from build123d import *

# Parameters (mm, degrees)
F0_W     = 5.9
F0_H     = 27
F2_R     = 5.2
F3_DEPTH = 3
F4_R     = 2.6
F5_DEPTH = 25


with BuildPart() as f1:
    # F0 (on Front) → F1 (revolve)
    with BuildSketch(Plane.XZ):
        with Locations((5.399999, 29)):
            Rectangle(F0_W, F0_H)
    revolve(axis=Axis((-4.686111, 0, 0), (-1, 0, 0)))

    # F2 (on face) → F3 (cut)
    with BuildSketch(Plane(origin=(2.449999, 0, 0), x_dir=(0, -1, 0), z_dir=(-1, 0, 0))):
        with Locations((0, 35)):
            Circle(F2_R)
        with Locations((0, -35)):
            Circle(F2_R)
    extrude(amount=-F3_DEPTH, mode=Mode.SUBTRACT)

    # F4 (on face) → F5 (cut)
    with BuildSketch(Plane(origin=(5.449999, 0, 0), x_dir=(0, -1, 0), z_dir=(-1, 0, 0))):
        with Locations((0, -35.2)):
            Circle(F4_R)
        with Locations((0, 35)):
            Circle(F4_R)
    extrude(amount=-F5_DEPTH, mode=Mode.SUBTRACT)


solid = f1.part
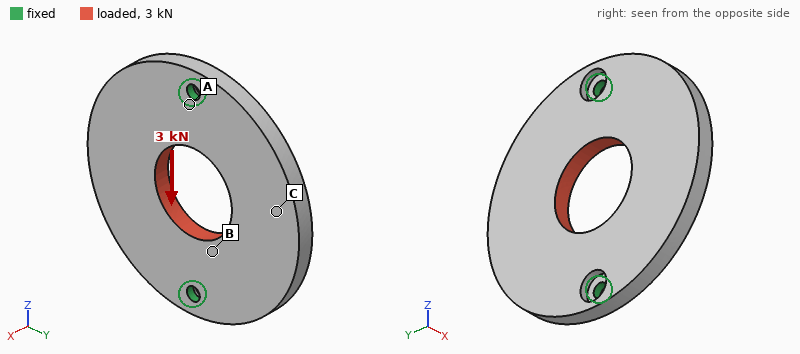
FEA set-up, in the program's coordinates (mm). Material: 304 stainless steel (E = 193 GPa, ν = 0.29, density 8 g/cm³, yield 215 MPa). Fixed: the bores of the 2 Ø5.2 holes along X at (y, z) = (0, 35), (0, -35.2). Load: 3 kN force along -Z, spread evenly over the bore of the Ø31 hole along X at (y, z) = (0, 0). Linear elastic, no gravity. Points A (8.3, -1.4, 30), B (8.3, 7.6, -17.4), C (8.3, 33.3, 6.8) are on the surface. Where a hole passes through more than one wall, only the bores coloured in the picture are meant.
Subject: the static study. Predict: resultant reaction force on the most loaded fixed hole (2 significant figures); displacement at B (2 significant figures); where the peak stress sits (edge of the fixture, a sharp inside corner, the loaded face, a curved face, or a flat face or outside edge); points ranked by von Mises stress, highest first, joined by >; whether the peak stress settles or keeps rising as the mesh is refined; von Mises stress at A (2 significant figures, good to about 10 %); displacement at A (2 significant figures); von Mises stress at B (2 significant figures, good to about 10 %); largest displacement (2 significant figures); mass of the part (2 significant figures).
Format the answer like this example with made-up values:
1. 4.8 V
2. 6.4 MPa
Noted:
1. 1.5 kN
2. 2.0 µm
3. edge of the fixture
4. A > B > C
5. keeps rising
6. 28 MPa
7. 0.42 µm
8. 12 MPa
9. 2.7 µm
10. 230 g
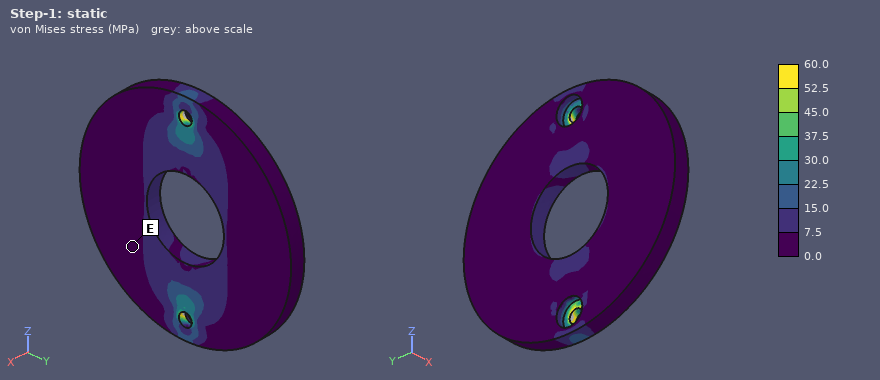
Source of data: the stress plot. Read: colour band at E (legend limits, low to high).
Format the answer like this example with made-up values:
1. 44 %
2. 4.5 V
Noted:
1. 0.0 to 7.5 MPa
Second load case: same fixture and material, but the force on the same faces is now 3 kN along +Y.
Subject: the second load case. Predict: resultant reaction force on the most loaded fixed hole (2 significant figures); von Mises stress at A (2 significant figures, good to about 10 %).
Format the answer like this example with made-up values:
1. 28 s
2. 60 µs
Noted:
1. 1.5 kN
2. 9.2 MPa
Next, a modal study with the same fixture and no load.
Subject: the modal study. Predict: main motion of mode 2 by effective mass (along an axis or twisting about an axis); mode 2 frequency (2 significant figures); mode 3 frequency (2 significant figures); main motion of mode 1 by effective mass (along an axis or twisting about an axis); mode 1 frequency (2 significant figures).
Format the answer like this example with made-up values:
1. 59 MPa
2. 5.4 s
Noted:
1. along X
2. 2200 Hz
3. 4700 Hz
4. twisting about Z
5. 1400 Hz
